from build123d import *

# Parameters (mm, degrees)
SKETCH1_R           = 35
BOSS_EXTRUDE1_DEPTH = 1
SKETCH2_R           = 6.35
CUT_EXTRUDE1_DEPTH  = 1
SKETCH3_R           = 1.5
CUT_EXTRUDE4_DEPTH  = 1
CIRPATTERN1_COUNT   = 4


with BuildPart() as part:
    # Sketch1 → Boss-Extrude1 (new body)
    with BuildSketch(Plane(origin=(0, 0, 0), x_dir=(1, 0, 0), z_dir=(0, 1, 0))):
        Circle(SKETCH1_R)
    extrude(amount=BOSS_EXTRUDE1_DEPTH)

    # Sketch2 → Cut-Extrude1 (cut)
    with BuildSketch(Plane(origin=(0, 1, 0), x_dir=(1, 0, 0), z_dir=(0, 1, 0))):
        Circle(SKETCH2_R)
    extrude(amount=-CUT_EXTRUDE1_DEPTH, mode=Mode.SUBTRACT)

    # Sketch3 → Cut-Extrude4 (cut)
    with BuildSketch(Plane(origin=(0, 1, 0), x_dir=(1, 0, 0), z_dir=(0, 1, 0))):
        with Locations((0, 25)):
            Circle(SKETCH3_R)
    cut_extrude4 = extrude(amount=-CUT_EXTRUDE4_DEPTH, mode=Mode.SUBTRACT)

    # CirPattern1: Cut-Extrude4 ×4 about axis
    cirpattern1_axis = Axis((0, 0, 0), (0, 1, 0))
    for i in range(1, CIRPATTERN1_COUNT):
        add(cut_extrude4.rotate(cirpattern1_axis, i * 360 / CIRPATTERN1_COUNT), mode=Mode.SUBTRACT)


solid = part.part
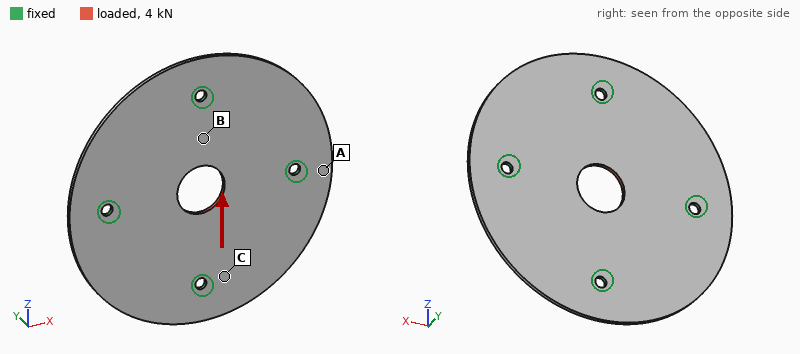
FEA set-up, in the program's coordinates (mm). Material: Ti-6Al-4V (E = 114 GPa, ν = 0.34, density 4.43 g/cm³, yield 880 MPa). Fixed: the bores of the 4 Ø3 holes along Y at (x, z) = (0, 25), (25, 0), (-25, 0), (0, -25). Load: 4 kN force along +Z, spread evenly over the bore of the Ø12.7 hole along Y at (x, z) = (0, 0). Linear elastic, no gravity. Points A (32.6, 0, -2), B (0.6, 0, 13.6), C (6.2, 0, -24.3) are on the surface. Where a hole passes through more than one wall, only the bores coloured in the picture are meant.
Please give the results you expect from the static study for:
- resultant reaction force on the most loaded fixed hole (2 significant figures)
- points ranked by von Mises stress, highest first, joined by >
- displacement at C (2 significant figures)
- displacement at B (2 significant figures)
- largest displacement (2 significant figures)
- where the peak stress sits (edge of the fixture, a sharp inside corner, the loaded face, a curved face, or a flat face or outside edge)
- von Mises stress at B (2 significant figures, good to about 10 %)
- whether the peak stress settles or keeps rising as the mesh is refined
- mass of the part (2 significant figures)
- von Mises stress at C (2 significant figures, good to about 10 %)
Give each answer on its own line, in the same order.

1.3 kN
B > C > A
5.5 µm
11 µm
19 µm
edge of the fixture
100 MPa
keeps rising
16 g
42 MPa
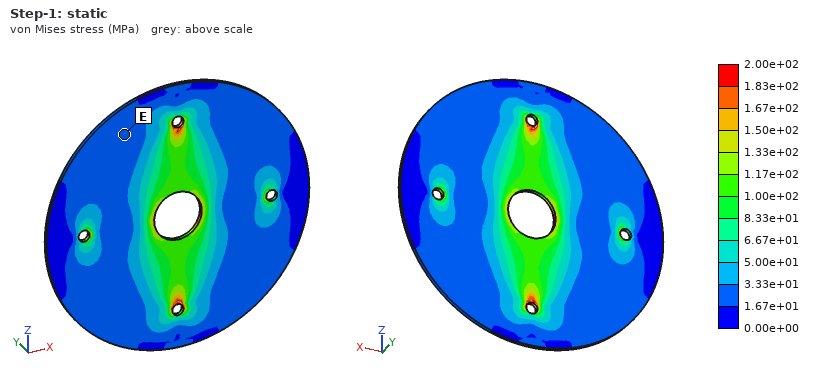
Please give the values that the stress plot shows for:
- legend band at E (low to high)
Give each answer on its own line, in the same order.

1.67e+01 to 3.33e+01 MPa
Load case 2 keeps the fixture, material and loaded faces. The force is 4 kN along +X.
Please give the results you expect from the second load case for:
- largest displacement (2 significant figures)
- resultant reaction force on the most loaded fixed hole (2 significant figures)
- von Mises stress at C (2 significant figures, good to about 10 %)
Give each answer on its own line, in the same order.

19 µm
1.3 kN
41 MPa
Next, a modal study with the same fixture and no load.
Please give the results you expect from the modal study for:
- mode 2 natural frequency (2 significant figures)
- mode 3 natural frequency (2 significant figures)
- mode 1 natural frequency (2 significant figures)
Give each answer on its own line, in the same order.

2600 Hz
2600 Hz
2500 Hz
